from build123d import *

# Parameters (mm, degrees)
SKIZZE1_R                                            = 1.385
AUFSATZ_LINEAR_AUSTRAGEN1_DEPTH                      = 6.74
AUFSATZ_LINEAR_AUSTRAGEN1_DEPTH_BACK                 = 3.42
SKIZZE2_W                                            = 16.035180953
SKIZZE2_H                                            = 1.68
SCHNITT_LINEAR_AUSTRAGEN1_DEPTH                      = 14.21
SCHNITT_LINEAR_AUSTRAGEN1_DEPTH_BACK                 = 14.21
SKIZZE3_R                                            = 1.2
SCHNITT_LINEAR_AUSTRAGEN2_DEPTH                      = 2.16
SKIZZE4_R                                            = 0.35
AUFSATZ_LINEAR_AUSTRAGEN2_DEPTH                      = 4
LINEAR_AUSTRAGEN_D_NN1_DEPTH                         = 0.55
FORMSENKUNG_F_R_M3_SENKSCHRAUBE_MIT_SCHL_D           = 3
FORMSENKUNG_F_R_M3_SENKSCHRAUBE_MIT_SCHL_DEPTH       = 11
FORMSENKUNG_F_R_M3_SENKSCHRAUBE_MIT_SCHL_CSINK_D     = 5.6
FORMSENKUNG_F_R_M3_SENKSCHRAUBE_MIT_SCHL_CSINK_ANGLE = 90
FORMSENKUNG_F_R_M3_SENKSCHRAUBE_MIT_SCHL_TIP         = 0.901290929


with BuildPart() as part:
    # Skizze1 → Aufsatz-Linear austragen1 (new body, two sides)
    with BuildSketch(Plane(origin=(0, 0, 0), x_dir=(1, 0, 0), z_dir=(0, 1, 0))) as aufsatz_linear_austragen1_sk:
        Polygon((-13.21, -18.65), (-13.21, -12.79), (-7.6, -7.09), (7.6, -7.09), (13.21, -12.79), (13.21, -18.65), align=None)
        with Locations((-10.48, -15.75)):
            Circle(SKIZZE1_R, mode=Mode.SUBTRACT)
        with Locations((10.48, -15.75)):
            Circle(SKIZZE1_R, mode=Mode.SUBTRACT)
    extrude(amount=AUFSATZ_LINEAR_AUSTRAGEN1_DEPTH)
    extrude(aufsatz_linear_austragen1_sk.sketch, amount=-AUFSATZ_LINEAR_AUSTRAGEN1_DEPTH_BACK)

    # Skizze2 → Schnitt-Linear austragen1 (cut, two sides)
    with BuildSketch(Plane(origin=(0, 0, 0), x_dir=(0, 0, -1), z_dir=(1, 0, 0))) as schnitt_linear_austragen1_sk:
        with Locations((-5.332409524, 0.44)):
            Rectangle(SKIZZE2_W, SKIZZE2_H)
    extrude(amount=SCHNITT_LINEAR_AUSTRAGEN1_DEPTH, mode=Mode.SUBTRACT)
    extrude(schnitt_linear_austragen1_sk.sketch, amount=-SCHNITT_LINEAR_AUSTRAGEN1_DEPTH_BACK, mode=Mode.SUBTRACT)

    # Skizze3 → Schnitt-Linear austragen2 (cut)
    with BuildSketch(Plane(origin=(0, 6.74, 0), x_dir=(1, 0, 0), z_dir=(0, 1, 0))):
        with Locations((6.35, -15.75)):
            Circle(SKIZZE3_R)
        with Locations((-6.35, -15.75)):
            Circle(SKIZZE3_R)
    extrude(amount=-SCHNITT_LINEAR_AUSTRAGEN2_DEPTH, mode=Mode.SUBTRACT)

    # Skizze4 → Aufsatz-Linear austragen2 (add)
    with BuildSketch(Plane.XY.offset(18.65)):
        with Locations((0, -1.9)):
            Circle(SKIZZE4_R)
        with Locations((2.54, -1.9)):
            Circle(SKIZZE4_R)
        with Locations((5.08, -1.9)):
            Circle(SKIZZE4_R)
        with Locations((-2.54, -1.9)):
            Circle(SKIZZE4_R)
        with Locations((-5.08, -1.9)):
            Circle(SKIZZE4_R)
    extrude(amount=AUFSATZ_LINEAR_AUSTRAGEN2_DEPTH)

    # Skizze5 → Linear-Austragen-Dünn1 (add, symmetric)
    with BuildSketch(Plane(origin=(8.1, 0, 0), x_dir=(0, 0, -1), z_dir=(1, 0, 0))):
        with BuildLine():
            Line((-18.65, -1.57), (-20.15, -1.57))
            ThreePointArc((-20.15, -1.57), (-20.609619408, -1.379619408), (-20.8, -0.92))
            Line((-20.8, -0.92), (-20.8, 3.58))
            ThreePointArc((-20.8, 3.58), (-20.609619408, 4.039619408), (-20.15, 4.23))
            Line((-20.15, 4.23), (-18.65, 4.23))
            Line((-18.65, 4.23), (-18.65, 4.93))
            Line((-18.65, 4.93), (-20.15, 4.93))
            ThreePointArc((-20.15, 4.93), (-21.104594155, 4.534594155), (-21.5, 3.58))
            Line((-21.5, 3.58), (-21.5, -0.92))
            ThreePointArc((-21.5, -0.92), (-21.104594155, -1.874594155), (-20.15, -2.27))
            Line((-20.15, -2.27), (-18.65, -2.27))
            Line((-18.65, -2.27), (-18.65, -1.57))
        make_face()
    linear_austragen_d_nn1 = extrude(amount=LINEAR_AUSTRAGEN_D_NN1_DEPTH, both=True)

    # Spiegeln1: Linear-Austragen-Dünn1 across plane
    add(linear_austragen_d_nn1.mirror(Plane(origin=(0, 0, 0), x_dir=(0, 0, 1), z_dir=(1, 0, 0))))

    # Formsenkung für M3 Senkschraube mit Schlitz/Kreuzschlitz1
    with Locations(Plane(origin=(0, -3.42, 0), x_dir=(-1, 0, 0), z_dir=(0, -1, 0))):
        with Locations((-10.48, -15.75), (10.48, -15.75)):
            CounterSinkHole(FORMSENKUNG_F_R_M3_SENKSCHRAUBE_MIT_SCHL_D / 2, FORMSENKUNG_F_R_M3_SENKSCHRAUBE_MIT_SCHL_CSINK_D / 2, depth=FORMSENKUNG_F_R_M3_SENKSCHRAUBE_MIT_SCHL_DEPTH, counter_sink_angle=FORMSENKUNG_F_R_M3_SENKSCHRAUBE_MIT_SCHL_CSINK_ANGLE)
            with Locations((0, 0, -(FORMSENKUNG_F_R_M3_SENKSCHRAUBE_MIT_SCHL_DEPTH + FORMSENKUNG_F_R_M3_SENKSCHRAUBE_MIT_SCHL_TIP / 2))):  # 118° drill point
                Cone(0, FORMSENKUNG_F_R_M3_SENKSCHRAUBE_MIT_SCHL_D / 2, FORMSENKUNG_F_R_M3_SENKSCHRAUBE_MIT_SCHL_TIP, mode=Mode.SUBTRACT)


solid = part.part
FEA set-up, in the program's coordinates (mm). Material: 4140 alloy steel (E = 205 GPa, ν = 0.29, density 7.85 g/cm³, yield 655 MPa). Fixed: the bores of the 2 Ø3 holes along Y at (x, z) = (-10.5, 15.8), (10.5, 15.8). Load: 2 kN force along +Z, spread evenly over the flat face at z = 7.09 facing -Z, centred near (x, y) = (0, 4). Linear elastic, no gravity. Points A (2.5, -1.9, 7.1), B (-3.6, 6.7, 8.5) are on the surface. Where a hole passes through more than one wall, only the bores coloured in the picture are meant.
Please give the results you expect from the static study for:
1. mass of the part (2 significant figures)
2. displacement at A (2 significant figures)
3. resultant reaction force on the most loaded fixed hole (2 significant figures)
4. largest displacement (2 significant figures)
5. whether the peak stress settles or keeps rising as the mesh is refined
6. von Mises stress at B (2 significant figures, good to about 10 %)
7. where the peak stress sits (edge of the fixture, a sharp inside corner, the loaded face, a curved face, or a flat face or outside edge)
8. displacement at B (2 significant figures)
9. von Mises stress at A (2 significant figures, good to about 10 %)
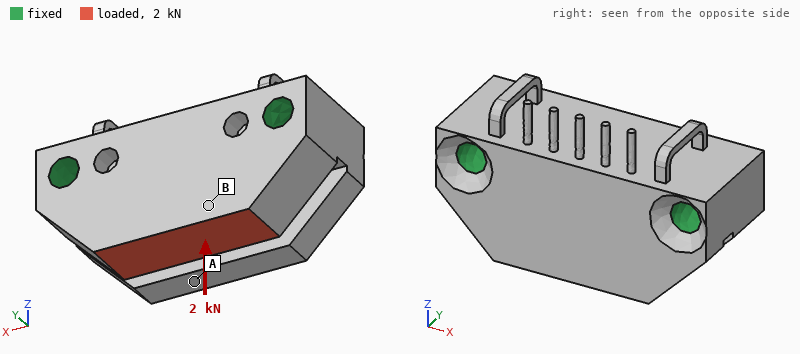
19 g
1.1 µm
1.1 kN
3.1 µm
keeps rising
22 MPa
edge of the fixture
2.6 µm
9.3 MPa
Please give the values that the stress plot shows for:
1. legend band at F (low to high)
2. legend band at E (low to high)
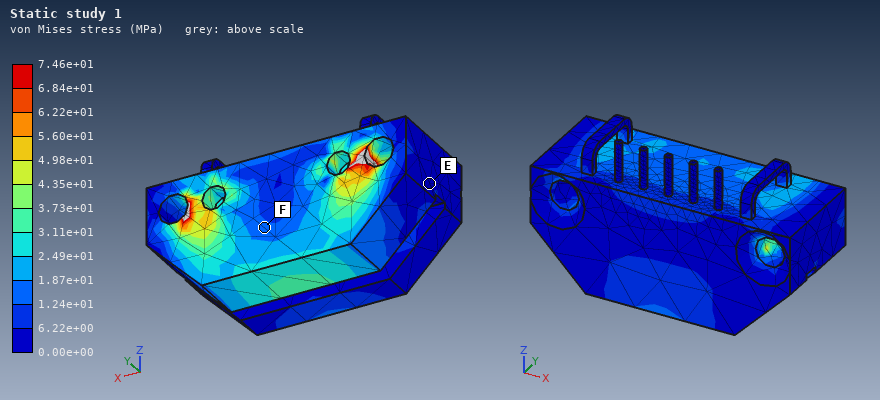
1.24e+01 to 1.87e+01 MPa
0.00e+00 to 6.22e+00 MPa
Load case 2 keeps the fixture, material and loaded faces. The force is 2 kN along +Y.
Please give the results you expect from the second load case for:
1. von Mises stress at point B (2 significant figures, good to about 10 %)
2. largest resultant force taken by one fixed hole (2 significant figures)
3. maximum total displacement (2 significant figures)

55 MPa
1.0 kN
15 µm
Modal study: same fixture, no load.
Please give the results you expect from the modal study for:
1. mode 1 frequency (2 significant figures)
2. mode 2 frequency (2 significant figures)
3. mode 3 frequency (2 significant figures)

29 kHz
29 kHz
29 kHz
